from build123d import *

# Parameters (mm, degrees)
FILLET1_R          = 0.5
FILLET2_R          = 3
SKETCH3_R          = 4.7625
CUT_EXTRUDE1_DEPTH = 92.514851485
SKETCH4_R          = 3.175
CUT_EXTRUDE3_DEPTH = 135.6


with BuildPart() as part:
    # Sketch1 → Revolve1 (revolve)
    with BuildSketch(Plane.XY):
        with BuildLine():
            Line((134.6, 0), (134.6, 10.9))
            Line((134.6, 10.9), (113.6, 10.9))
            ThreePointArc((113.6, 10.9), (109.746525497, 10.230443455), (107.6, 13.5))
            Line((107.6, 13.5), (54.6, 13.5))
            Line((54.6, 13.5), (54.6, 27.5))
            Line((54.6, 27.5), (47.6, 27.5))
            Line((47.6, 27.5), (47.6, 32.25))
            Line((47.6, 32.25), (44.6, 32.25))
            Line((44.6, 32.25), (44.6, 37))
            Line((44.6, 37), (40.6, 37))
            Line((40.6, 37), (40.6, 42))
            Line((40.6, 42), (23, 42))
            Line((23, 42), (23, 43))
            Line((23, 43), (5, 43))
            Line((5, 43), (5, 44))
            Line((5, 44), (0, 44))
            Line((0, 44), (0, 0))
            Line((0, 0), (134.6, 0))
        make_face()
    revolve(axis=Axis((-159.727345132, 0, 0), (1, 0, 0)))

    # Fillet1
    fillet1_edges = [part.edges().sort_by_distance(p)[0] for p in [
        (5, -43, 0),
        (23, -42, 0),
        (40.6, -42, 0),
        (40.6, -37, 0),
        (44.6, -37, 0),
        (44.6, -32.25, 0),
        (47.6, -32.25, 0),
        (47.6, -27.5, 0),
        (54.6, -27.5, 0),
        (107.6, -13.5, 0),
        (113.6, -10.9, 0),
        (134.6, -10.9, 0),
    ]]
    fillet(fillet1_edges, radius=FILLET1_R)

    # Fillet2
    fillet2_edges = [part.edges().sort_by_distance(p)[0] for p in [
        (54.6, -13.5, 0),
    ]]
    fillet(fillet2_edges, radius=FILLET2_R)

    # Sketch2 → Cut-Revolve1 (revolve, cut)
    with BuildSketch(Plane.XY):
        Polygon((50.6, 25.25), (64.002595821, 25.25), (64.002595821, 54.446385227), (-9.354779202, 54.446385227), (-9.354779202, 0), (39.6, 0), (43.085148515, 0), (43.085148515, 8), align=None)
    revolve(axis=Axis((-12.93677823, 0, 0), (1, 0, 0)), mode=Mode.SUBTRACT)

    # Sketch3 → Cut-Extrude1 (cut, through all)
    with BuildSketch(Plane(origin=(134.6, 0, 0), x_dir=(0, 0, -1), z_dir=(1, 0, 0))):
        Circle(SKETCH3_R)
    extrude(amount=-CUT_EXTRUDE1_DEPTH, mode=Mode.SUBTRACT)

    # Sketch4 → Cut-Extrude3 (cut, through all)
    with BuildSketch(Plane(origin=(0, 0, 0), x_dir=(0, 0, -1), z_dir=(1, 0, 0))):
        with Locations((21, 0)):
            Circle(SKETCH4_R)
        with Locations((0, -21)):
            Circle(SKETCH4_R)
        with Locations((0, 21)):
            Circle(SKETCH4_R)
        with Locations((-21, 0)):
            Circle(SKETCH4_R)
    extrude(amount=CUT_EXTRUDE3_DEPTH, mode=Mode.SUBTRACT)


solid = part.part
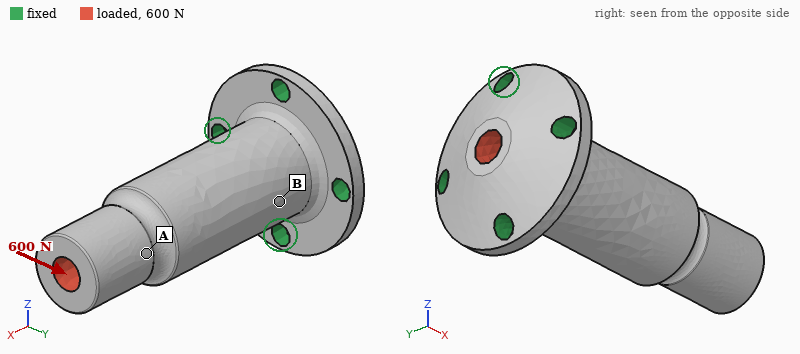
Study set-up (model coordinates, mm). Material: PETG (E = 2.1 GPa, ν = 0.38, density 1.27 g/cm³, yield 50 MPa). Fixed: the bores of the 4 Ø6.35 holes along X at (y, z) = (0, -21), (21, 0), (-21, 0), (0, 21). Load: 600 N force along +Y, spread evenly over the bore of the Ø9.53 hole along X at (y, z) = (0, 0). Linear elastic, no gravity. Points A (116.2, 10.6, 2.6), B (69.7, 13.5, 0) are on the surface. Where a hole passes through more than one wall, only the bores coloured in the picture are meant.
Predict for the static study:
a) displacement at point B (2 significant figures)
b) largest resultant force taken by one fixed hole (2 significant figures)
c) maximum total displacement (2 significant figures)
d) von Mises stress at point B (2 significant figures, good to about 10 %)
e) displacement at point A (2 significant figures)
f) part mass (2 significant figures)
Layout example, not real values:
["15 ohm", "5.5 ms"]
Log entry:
["0.19 mm", "630 N", "1.1 mm", "7.2 MPa", "0.78 mm", "61 g"]
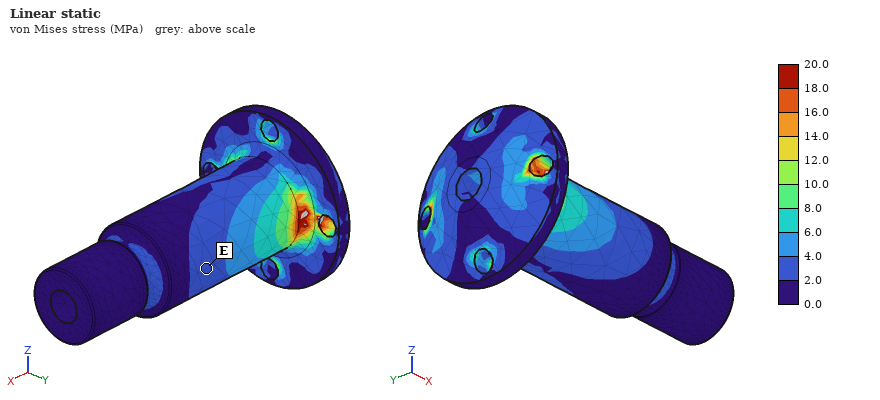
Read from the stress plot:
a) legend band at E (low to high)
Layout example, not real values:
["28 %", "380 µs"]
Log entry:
["2.0 to 4.0 MPa"]
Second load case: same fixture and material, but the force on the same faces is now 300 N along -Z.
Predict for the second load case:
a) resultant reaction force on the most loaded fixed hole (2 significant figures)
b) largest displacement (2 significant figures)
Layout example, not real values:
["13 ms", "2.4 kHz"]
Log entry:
["310 N", "0.53 mm"]
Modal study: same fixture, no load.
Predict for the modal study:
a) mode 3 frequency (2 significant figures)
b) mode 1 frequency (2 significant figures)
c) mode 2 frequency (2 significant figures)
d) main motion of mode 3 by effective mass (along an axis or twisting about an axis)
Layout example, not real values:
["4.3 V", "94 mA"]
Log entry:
["2800 Hz", "740 Hz", "740 Hz", "twisting about X"]
